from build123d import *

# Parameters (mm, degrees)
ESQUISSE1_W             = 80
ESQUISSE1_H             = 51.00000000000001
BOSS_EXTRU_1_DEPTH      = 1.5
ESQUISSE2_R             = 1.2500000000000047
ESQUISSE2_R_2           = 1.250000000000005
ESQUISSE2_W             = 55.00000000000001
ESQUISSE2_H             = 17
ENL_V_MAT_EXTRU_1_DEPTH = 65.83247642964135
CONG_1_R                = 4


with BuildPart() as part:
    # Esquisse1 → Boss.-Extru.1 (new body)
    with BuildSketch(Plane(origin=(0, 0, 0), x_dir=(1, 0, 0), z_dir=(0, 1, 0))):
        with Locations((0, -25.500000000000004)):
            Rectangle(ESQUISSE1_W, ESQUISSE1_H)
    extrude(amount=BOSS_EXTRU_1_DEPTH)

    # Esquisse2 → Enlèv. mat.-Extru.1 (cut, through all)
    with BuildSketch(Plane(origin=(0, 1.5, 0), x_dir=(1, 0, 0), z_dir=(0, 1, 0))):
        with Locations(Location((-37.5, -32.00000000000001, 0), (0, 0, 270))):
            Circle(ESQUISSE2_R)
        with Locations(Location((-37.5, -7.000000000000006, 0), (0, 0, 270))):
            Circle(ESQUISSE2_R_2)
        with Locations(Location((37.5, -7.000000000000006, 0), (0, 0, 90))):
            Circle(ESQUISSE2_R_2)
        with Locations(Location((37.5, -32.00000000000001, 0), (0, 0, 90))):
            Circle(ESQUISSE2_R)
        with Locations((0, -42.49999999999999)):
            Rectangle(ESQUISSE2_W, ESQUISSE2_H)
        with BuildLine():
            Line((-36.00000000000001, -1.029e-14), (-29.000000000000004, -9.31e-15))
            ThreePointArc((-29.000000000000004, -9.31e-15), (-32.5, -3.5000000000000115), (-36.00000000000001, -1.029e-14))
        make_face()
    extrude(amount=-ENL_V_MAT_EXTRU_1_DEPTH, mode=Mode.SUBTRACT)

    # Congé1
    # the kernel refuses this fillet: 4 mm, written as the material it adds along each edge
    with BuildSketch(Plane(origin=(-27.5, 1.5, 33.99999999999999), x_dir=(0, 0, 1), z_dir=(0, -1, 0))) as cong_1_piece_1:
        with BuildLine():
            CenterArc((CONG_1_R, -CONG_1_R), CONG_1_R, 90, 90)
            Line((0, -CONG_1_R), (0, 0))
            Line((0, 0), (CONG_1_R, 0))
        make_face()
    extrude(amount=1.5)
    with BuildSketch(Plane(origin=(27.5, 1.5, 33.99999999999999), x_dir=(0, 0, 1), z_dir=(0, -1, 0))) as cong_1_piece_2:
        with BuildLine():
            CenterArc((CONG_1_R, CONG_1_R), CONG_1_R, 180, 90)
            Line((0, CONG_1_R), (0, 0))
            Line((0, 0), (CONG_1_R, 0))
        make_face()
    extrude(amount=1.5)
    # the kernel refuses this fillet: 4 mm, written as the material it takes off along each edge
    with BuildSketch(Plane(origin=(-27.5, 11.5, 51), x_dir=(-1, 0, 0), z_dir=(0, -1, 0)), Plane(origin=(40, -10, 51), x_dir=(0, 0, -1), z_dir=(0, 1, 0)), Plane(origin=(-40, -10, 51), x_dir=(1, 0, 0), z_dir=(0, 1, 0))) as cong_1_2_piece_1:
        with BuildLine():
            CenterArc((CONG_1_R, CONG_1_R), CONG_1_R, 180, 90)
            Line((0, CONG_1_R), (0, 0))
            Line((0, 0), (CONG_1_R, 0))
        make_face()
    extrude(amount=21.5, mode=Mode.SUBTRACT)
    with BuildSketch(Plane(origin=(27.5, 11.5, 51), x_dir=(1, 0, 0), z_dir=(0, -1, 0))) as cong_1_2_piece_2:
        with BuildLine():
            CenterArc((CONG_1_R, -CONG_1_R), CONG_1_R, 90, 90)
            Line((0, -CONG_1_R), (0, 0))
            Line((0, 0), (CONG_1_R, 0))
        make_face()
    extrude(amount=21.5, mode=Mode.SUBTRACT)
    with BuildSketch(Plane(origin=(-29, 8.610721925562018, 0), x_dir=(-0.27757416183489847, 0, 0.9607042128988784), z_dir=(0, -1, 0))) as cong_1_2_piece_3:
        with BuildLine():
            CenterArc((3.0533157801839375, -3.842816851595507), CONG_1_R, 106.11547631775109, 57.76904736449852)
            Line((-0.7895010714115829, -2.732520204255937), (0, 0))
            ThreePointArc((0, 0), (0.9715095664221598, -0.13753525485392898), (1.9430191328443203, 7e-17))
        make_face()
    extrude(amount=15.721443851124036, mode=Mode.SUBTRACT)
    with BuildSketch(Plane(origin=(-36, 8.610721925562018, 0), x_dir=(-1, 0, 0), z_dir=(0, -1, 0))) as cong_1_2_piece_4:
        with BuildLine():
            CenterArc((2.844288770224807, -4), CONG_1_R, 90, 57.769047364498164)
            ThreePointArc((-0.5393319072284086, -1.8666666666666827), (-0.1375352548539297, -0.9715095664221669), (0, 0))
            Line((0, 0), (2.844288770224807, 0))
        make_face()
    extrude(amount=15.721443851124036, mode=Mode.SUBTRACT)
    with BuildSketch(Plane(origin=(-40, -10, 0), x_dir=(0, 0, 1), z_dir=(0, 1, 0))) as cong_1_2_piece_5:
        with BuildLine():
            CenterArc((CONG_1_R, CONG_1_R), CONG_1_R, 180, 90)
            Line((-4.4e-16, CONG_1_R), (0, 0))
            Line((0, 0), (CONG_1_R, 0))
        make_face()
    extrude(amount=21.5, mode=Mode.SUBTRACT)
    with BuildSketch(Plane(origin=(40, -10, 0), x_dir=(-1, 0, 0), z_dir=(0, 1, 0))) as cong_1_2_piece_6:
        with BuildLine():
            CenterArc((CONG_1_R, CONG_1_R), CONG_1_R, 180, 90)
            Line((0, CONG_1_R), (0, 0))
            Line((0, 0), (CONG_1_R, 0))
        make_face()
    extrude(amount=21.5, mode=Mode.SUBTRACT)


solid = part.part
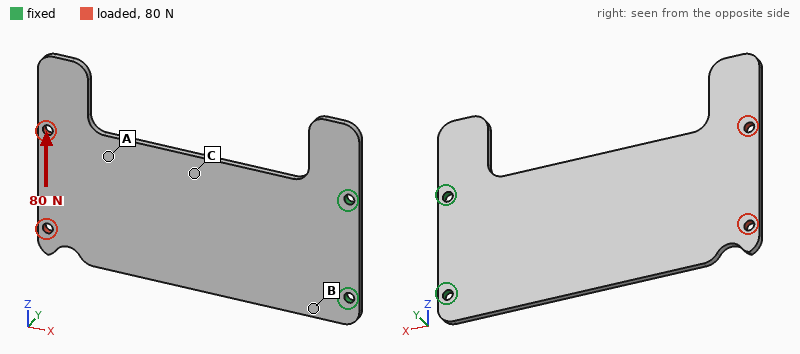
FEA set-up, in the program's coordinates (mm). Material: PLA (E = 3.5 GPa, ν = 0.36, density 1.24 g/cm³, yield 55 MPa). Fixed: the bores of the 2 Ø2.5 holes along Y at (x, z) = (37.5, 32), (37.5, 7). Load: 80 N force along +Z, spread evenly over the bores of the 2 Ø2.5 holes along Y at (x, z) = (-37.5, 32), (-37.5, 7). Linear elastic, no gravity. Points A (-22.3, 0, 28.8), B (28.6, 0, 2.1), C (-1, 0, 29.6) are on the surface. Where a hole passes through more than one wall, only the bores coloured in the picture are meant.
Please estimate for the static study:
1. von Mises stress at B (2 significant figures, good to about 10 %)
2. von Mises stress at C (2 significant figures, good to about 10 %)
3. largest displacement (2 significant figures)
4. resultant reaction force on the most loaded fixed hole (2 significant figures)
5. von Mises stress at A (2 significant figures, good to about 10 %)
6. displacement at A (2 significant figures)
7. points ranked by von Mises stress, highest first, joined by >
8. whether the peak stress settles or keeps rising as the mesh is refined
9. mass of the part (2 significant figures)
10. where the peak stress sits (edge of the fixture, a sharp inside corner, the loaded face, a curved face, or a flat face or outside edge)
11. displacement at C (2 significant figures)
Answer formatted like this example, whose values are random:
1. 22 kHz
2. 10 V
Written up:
1. 12 MPa
2. 7.7 MPa
3. 0.97 mm
4. 240 N
5. 3.3 MPa
6. 0.61 mm
7. B > C > A
8. keeps rising
9. 5.7 g
10. edge of the fixture
11. 0.33 mm
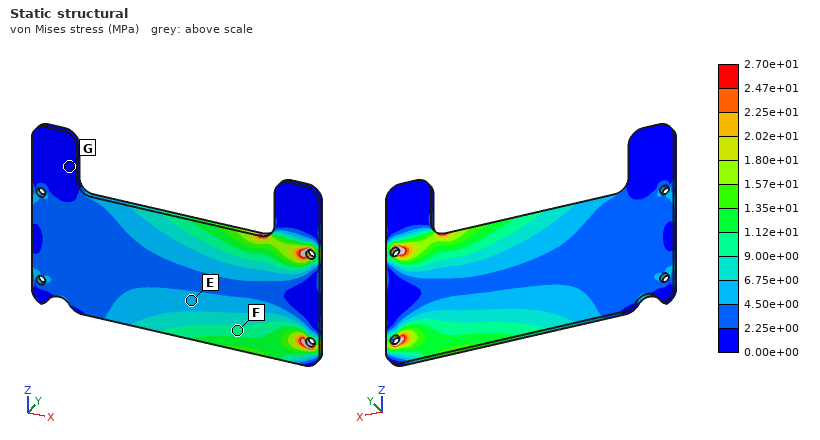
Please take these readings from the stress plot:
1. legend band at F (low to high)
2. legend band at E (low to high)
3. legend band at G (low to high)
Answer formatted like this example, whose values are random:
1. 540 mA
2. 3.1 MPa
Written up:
1. 9.00e+00 to 1.12e+01 MPa
2. 4.50e+00 to 6.75e+00 MPa
3. 0.00e+00 to 2.25e+00 MPa
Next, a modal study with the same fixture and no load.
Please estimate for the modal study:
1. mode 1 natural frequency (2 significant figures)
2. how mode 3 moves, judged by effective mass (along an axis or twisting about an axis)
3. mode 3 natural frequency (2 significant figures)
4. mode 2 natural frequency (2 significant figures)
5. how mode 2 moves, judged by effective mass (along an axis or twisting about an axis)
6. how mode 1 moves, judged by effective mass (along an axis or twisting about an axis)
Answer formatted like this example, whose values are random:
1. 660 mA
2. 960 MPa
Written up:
1. 61 Hz
2. along Y
3. 430 Hz
4. 230 Hz
5. twisting about X
6. along Y
